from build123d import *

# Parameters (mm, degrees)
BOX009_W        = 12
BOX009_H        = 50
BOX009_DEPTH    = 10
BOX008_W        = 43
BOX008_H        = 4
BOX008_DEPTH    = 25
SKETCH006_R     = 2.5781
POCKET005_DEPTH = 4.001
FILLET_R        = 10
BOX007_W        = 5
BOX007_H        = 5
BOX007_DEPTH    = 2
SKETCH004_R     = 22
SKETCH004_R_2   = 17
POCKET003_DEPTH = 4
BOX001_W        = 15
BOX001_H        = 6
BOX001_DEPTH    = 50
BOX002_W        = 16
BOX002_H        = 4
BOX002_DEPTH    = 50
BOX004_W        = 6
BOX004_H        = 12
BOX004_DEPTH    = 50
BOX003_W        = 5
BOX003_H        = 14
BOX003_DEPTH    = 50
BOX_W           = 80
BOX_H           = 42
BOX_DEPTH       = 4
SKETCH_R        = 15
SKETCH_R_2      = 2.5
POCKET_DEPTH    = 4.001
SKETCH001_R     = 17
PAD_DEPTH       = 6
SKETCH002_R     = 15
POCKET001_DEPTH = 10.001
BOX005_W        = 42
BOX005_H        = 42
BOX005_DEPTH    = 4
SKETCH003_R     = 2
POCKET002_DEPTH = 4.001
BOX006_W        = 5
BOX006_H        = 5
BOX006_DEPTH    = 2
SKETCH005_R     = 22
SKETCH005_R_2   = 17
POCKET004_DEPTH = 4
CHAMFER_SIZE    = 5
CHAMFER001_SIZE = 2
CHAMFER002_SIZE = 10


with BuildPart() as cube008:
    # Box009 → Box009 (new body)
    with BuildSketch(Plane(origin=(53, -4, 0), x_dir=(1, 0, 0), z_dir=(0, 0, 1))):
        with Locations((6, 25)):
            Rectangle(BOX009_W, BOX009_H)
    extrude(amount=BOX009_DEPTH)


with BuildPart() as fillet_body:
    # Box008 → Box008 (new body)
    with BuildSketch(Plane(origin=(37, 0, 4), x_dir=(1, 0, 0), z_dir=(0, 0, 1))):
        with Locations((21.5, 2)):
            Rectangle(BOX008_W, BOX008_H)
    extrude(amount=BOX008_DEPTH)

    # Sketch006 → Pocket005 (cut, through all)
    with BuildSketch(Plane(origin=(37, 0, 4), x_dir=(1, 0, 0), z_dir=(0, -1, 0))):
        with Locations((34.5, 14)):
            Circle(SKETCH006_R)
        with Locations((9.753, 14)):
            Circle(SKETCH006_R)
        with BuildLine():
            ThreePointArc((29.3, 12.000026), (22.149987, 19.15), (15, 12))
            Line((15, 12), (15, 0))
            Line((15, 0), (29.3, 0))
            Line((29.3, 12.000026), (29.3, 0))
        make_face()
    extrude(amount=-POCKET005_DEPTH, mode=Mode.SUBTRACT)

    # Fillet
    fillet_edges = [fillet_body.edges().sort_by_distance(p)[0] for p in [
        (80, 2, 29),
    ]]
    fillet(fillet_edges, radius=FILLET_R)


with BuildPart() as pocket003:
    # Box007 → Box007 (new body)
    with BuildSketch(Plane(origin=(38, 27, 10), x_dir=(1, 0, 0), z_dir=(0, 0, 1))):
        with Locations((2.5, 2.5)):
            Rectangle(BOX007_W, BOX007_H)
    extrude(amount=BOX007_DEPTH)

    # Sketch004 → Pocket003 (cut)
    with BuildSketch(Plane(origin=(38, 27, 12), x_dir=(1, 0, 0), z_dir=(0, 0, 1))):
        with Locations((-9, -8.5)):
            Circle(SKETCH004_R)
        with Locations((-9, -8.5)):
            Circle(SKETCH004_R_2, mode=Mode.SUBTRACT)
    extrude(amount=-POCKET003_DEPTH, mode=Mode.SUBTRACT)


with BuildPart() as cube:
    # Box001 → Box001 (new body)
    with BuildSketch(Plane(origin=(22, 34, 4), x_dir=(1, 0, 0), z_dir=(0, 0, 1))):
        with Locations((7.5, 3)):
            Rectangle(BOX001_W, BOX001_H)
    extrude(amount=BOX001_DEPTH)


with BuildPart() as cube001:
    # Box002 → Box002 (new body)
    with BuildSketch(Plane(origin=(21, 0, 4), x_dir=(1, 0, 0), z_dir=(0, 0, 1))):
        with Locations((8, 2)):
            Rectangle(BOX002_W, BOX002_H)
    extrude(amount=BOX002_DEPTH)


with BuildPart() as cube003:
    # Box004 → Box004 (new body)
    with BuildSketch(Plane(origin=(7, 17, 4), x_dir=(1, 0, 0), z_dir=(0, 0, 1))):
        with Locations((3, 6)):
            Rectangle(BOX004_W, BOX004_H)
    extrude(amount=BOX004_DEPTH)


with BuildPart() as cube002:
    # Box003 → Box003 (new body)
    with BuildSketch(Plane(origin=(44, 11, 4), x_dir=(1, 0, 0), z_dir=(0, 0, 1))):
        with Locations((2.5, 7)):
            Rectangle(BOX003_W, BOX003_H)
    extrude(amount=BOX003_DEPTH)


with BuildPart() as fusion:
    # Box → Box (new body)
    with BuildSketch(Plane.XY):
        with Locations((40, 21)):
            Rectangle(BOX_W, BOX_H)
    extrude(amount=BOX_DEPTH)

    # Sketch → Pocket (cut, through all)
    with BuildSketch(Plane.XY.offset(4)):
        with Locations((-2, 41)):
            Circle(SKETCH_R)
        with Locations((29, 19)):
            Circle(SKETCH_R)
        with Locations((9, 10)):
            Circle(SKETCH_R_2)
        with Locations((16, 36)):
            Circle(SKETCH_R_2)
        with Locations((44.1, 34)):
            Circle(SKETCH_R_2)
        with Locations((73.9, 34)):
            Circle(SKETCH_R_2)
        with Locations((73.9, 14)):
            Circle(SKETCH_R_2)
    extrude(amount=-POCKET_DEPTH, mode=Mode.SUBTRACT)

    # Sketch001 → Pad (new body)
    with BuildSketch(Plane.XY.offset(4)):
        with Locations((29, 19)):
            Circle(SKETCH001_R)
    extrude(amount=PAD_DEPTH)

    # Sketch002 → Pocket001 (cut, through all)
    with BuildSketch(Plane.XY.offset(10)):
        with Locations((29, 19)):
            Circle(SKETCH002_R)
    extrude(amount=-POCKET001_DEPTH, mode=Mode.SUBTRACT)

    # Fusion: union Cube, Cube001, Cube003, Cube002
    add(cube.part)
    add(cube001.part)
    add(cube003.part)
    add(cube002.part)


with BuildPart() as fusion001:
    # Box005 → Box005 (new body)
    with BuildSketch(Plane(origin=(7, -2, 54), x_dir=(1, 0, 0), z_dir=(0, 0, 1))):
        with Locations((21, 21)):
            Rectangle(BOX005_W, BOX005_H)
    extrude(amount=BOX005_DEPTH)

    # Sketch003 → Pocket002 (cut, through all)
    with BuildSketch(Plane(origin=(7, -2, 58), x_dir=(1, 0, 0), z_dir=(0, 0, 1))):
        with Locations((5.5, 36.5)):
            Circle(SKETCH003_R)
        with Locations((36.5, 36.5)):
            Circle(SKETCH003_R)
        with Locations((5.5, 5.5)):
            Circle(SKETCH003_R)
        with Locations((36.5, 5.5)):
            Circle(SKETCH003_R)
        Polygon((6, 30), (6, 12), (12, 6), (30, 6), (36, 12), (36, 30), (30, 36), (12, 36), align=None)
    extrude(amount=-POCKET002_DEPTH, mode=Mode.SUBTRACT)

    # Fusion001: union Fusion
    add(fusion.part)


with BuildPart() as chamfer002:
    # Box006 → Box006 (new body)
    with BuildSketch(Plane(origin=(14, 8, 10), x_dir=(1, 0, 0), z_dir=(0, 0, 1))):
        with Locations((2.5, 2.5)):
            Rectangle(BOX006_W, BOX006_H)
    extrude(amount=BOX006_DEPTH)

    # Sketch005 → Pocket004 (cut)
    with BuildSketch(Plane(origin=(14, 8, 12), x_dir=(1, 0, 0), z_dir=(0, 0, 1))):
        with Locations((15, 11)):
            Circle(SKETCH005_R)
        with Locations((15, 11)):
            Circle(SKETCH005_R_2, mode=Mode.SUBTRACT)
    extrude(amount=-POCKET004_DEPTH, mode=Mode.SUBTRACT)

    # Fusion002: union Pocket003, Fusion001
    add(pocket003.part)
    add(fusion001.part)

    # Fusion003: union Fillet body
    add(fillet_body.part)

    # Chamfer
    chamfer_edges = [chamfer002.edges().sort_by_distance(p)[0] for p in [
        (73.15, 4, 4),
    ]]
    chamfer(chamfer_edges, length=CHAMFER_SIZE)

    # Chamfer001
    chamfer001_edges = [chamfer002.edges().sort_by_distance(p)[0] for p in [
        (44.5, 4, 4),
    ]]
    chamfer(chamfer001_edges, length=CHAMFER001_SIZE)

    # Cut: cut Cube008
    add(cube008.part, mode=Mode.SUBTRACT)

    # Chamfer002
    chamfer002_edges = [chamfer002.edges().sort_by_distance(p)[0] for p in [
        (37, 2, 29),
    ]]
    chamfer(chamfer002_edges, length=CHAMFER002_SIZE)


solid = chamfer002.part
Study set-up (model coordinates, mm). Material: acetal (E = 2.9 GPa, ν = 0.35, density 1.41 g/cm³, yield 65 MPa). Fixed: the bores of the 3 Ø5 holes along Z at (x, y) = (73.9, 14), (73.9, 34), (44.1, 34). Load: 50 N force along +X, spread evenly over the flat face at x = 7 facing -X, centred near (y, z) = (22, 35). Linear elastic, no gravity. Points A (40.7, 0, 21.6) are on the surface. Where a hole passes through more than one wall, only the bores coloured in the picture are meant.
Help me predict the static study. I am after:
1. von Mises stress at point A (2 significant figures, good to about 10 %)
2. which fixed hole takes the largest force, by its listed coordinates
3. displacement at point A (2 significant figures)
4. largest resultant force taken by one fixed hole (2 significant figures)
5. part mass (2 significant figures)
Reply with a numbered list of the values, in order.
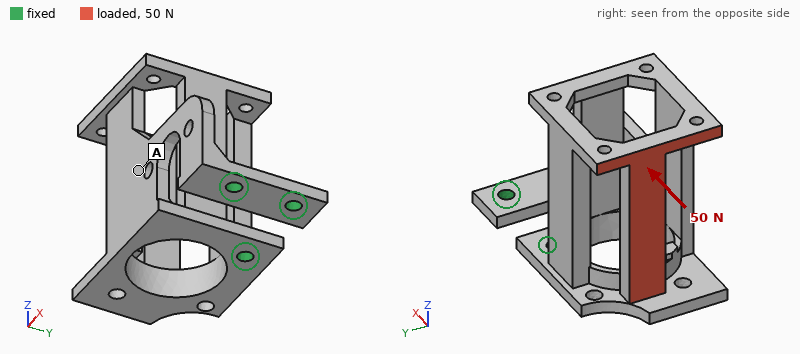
1. 1.5 MPa
2. (73.9, 14)
3. 0.40 mm
4. 41 N
5. 43 g
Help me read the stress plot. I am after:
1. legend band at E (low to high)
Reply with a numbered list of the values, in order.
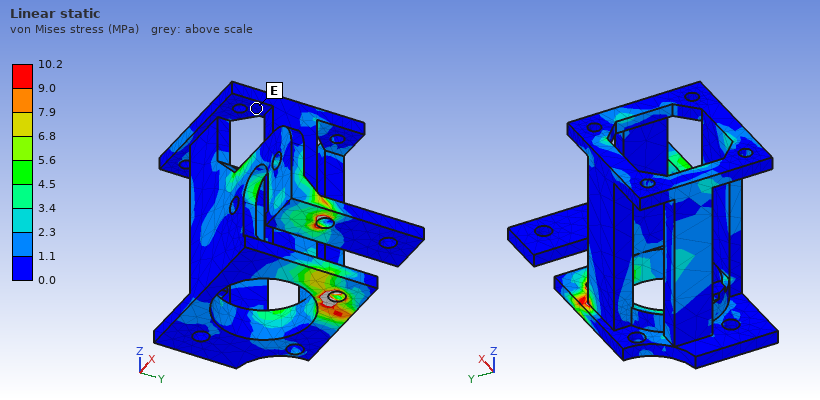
1. 0.0 to 1.1 MPa
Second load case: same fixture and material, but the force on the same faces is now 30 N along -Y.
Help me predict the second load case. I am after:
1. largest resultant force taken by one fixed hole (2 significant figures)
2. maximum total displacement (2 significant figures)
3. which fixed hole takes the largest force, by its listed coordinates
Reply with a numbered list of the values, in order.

1. 33 N
2. 1.1 mm
3. (44.1, 34)
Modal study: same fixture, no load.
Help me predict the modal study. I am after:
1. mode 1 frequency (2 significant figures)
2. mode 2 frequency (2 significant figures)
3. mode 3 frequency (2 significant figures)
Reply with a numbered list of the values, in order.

1. 170 Hz
2. 420 Hz
3. 540 Hz
